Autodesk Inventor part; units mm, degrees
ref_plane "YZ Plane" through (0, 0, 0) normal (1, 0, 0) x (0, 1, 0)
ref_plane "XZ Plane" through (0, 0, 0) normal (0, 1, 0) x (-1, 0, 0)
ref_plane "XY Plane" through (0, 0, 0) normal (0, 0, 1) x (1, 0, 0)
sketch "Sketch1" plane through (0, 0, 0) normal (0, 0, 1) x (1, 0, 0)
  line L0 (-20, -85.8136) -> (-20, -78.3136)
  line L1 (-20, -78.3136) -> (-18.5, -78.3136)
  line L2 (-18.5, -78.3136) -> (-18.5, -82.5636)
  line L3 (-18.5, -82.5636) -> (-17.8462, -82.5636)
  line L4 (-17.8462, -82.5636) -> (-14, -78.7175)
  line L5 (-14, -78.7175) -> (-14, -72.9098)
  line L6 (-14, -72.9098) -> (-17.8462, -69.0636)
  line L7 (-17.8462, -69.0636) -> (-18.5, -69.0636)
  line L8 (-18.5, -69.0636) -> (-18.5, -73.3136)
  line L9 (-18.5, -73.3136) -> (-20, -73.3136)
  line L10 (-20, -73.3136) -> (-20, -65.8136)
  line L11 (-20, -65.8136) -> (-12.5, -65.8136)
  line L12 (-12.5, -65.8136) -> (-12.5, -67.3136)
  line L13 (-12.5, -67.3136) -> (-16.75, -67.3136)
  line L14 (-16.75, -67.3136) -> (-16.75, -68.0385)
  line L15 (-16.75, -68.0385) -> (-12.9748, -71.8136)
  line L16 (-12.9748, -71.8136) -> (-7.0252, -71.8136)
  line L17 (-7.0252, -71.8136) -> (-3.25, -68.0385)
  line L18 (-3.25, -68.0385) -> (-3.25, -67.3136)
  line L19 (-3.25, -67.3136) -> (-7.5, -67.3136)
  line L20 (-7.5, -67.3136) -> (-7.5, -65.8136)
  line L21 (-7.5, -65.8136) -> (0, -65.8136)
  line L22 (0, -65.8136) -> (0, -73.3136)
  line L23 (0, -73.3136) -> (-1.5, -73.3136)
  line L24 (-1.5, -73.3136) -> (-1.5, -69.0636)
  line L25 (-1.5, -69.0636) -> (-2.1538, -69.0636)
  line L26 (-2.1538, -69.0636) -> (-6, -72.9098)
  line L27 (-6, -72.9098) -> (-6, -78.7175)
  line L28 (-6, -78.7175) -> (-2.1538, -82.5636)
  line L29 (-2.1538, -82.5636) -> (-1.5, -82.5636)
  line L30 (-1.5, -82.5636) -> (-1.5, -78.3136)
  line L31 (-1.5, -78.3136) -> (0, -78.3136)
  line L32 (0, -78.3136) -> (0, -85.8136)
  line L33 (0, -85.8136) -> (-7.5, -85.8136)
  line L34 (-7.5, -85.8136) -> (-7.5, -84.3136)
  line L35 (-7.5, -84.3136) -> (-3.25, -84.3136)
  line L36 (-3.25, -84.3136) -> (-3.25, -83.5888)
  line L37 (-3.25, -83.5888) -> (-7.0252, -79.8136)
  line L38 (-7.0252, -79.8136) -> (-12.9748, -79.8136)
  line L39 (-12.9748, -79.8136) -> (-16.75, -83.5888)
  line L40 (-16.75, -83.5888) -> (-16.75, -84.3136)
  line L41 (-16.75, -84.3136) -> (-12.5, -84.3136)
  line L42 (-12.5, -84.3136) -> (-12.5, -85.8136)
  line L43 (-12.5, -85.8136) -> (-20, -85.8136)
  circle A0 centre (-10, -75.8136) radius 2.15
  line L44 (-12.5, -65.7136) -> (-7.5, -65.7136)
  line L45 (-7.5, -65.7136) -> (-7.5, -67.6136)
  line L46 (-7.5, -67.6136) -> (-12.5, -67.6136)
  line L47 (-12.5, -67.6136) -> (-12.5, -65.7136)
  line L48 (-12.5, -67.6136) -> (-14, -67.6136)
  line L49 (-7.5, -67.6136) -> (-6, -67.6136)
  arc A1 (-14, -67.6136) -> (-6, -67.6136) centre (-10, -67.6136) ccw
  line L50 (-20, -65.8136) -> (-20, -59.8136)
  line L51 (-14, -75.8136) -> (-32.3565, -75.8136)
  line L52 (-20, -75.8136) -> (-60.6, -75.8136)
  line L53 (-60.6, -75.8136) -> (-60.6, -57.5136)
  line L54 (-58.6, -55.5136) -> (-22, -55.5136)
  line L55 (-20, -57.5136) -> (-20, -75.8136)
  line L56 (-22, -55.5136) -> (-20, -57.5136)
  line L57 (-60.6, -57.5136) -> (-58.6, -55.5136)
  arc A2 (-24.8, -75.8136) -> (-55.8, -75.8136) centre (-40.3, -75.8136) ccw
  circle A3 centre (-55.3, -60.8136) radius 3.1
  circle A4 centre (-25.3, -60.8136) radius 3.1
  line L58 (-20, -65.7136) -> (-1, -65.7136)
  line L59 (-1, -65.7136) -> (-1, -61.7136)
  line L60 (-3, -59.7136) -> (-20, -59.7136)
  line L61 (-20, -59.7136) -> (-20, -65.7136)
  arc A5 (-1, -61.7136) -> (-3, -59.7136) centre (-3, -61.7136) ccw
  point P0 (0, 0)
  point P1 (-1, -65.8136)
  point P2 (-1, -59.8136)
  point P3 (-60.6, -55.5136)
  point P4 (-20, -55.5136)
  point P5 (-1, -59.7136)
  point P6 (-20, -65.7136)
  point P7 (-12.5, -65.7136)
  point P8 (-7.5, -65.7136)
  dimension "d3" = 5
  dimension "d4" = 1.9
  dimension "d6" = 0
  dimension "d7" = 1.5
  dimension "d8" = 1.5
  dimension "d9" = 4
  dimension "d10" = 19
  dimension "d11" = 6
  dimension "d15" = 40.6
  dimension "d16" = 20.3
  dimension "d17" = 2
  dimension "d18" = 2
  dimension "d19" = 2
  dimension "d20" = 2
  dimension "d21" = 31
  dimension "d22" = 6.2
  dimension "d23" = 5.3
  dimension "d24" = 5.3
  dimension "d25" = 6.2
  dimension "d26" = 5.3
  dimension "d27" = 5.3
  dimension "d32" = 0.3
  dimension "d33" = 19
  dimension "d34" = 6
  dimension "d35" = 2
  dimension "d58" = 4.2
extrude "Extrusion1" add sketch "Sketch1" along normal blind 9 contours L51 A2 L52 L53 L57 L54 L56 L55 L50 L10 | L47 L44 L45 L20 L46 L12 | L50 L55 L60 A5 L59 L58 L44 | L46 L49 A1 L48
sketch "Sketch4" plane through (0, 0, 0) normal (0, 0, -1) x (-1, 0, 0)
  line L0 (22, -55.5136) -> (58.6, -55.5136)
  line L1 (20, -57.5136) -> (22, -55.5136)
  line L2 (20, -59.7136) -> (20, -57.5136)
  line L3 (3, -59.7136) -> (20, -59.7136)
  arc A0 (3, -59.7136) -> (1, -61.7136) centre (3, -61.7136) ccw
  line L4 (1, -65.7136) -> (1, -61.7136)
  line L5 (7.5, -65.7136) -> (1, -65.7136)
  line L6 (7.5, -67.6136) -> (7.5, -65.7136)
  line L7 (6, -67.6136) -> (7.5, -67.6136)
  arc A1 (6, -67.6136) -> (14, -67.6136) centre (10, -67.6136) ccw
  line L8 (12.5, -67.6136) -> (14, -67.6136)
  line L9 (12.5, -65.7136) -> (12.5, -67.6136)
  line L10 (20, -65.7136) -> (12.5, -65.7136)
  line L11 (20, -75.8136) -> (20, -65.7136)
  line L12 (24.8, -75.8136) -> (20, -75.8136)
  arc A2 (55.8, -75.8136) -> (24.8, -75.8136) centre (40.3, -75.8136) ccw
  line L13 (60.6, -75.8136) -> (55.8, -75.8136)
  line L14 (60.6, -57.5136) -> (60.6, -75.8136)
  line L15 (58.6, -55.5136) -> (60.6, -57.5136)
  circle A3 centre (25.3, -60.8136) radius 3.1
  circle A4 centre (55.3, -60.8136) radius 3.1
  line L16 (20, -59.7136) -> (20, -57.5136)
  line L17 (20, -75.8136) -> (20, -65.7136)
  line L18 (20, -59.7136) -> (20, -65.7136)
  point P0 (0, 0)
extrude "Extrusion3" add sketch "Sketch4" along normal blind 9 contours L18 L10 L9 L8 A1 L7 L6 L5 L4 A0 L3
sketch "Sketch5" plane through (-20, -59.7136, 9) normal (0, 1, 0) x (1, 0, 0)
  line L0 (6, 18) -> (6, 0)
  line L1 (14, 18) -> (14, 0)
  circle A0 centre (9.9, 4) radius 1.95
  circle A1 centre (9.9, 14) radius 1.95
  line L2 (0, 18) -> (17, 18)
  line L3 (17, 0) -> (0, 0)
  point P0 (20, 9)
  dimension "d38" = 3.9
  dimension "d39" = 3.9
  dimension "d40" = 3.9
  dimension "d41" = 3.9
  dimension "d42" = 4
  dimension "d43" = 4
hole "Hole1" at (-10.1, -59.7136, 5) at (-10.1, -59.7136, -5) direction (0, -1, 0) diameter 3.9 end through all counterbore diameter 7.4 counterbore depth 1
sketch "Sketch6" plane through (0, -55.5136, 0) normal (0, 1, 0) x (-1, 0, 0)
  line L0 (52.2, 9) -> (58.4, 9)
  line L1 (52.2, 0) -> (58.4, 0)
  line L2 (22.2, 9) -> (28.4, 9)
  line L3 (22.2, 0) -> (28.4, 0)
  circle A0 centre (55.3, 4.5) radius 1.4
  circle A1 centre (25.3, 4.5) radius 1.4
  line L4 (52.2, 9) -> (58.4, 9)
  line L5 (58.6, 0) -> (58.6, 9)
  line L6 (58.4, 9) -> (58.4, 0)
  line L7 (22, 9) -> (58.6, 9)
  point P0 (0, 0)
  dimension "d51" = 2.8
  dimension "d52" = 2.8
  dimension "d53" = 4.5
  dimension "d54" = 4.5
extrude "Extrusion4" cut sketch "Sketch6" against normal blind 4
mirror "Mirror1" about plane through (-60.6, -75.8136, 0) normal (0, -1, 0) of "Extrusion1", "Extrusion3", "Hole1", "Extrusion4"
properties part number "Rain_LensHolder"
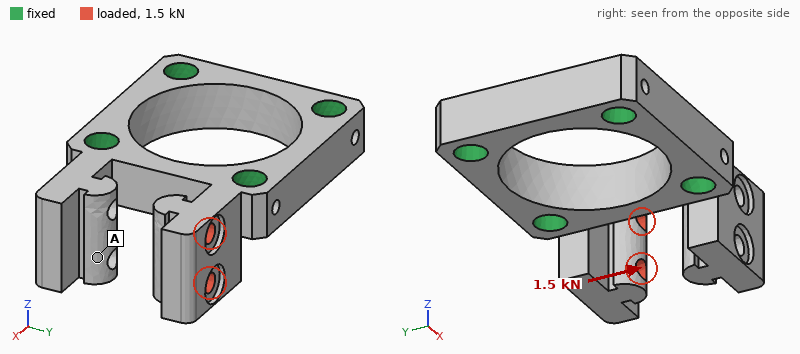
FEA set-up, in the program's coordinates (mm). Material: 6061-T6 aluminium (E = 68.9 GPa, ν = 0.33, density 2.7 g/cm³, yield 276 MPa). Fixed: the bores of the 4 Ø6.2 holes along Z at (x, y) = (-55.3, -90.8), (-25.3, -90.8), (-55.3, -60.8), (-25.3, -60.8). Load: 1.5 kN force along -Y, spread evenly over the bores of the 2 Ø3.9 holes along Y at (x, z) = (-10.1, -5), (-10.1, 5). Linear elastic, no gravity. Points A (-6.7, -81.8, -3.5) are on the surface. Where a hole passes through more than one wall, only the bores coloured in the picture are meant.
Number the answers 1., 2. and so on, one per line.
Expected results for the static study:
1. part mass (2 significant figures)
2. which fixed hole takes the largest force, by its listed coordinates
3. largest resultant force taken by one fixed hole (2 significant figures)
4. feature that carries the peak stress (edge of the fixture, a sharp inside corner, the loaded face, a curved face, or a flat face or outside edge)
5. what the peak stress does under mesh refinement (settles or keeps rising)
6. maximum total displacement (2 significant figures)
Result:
1. 31 g
2. (-25.3, -60.8)
3. 1.1 kN
4. a sharp inside corner
5. keeps rising
6. 0.20 mm
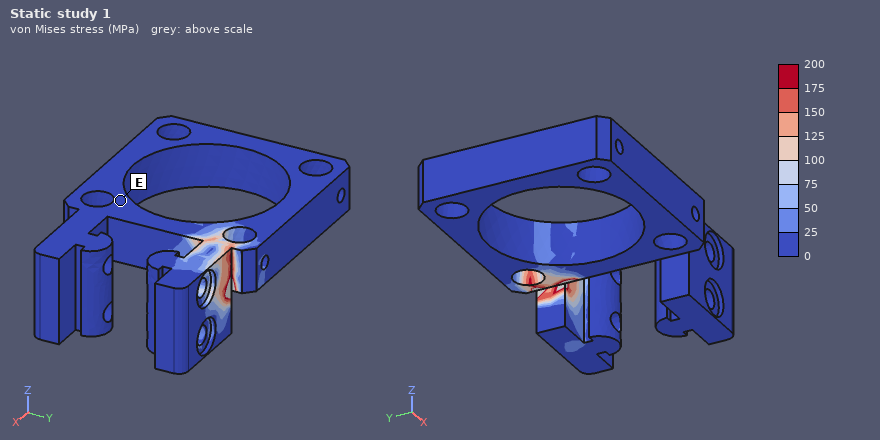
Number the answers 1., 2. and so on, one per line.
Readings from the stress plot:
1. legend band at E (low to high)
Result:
1. 0 to 25 MPa
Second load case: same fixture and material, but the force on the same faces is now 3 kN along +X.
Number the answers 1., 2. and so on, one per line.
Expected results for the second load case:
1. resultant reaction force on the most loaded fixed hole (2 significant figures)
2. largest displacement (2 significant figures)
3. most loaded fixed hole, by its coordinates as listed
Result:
1. 2.9 kN
2. 0.19 mm
3. (-25.3, -60.8)
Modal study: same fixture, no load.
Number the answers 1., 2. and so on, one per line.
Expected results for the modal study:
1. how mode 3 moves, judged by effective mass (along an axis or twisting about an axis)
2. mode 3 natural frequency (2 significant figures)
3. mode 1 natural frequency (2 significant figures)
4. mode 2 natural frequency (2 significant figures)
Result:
1. along Z
2. 9100 Hz
3. 7000 Hz
4. 7000 Hz
